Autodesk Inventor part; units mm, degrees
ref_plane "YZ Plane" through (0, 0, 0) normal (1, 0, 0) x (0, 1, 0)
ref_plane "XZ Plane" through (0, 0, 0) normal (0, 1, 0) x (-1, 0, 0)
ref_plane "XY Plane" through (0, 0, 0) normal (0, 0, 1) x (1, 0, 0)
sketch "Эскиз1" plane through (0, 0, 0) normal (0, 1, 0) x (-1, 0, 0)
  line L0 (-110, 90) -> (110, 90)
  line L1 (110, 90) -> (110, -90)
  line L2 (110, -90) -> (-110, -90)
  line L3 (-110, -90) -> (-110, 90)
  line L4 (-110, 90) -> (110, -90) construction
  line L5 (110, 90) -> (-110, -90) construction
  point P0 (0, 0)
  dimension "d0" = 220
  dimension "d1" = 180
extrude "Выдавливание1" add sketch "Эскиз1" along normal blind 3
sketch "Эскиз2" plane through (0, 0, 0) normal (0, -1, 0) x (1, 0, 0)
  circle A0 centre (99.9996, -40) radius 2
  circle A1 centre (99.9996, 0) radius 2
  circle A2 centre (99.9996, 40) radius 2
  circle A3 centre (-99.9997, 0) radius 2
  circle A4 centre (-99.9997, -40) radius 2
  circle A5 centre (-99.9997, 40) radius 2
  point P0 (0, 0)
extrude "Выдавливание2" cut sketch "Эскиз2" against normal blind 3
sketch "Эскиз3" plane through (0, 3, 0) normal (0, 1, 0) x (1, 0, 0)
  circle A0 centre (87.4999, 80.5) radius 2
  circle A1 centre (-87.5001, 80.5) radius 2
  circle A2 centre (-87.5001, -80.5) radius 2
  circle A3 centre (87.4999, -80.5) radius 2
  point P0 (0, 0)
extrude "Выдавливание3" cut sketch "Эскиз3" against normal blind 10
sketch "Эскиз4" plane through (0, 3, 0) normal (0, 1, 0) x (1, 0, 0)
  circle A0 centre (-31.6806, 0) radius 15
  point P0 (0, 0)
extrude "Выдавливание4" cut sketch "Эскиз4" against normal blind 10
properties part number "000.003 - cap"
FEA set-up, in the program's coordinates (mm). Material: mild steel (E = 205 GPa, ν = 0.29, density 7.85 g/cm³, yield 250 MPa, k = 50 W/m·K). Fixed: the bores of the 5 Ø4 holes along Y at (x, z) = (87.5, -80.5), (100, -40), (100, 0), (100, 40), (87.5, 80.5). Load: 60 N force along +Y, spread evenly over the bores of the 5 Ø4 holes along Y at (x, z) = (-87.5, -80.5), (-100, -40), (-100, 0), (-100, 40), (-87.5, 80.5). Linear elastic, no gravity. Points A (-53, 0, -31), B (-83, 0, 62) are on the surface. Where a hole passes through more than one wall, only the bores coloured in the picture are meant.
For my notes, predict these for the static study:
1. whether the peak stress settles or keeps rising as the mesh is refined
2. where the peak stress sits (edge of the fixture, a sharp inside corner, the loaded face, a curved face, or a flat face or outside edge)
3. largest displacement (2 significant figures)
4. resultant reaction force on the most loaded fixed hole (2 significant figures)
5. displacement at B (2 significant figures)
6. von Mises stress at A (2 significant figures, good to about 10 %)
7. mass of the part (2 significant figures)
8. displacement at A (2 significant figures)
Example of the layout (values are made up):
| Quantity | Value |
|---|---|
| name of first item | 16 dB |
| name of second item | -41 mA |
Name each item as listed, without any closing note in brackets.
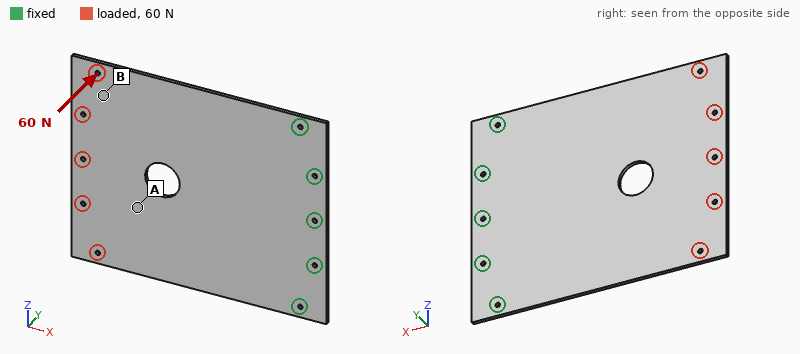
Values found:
| Quantity | Value |
|---|---|
| whether the peak stress settles or keeps rising as the mesh is refined | keeps rising |
| where the peak stress sits | edge of the fixture |
| largest displacement | 1.9 mm |
| resultant reaction force on the most loaded fixed hole | 30 N |
| displacement at B | 1.5 mm |
| von Mises stress at A | 10 MPa |
| mass of the part | 910 g |
| displacement at A | 1.1 mm |
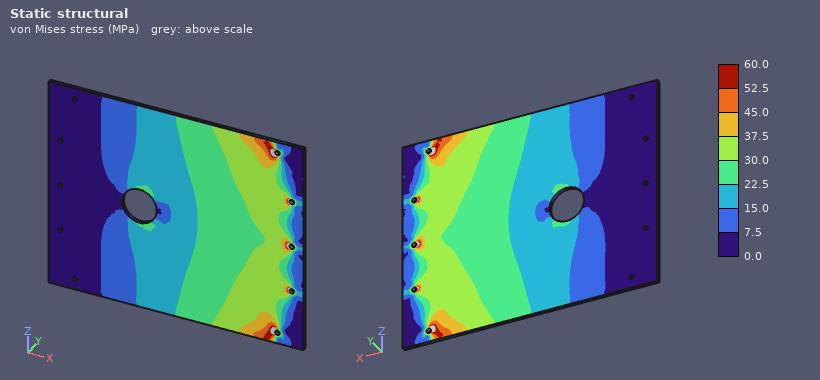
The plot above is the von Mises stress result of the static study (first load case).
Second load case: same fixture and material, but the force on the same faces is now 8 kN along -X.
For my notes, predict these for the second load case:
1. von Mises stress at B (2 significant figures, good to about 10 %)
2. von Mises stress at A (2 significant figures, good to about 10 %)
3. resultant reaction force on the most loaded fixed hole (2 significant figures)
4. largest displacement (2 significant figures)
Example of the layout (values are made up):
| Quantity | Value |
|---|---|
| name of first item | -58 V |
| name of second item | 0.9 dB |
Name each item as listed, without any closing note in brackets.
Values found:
| Quantity | Value |
|---|---|
| von Mises stress at B | 9.6 MPa |
| von Mises stress at A | 17 MPa |
| resultant reaction force on the most loaded fixed hole | 1.7 kN |
| largest displacement | 17 µm |
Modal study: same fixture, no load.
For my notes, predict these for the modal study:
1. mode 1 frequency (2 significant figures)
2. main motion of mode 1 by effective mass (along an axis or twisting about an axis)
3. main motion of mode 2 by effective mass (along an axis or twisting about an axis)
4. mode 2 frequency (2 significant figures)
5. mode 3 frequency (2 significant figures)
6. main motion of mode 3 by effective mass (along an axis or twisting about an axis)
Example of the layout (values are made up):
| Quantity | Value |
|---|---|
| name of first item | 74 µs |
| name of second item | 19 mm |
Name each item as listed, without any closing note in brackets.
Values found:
| Quantity | Value |
|---|---|
| mode 1 frequency | 60 Hz |
| main motion of mode 1 by effective mass | along Y |
| main motion of mode 2 by effective mass | twisting about X |
| mode 2 frequency | 170 Hz |
| mode 3 frequency | 370 Hz |
| main motion of mode 3 by effective mass | along Y |
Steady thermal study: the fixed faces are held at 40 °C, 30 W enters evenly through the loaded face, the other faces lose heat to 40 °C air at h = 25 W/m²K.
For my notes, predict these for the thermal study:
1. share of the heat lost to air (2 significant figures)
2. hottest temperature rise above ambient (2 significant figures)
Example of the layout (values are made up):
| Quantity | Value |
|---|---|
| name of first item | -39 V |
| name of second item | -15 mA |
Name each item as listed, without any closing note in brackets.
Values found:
| Quantity | Value |
|---|---|
| share of the heat lost to air | 96 % |
| hottest temperature rise above ambient | 57 K |
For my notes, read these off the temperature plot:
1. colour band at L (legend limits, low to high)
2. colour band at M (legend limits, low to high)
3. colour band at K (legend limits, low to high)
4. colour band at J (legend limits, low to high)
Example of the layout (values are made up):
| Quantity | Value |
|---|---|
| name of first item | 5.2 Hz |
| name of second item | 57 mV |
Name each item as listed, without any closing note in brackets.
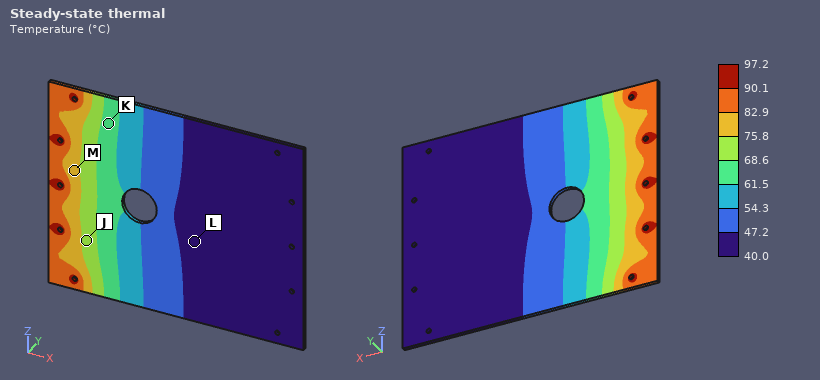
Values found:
| Quantity | Value |
|---|---|
| colour band at L | 40.0 to 47.2 °C |
| colour band at M | 75.8 to 82.9 °C |
| colour band at K | 61.5 to 68.6 °C |
| colour band at J | 68.6 to 75.8 °C |
